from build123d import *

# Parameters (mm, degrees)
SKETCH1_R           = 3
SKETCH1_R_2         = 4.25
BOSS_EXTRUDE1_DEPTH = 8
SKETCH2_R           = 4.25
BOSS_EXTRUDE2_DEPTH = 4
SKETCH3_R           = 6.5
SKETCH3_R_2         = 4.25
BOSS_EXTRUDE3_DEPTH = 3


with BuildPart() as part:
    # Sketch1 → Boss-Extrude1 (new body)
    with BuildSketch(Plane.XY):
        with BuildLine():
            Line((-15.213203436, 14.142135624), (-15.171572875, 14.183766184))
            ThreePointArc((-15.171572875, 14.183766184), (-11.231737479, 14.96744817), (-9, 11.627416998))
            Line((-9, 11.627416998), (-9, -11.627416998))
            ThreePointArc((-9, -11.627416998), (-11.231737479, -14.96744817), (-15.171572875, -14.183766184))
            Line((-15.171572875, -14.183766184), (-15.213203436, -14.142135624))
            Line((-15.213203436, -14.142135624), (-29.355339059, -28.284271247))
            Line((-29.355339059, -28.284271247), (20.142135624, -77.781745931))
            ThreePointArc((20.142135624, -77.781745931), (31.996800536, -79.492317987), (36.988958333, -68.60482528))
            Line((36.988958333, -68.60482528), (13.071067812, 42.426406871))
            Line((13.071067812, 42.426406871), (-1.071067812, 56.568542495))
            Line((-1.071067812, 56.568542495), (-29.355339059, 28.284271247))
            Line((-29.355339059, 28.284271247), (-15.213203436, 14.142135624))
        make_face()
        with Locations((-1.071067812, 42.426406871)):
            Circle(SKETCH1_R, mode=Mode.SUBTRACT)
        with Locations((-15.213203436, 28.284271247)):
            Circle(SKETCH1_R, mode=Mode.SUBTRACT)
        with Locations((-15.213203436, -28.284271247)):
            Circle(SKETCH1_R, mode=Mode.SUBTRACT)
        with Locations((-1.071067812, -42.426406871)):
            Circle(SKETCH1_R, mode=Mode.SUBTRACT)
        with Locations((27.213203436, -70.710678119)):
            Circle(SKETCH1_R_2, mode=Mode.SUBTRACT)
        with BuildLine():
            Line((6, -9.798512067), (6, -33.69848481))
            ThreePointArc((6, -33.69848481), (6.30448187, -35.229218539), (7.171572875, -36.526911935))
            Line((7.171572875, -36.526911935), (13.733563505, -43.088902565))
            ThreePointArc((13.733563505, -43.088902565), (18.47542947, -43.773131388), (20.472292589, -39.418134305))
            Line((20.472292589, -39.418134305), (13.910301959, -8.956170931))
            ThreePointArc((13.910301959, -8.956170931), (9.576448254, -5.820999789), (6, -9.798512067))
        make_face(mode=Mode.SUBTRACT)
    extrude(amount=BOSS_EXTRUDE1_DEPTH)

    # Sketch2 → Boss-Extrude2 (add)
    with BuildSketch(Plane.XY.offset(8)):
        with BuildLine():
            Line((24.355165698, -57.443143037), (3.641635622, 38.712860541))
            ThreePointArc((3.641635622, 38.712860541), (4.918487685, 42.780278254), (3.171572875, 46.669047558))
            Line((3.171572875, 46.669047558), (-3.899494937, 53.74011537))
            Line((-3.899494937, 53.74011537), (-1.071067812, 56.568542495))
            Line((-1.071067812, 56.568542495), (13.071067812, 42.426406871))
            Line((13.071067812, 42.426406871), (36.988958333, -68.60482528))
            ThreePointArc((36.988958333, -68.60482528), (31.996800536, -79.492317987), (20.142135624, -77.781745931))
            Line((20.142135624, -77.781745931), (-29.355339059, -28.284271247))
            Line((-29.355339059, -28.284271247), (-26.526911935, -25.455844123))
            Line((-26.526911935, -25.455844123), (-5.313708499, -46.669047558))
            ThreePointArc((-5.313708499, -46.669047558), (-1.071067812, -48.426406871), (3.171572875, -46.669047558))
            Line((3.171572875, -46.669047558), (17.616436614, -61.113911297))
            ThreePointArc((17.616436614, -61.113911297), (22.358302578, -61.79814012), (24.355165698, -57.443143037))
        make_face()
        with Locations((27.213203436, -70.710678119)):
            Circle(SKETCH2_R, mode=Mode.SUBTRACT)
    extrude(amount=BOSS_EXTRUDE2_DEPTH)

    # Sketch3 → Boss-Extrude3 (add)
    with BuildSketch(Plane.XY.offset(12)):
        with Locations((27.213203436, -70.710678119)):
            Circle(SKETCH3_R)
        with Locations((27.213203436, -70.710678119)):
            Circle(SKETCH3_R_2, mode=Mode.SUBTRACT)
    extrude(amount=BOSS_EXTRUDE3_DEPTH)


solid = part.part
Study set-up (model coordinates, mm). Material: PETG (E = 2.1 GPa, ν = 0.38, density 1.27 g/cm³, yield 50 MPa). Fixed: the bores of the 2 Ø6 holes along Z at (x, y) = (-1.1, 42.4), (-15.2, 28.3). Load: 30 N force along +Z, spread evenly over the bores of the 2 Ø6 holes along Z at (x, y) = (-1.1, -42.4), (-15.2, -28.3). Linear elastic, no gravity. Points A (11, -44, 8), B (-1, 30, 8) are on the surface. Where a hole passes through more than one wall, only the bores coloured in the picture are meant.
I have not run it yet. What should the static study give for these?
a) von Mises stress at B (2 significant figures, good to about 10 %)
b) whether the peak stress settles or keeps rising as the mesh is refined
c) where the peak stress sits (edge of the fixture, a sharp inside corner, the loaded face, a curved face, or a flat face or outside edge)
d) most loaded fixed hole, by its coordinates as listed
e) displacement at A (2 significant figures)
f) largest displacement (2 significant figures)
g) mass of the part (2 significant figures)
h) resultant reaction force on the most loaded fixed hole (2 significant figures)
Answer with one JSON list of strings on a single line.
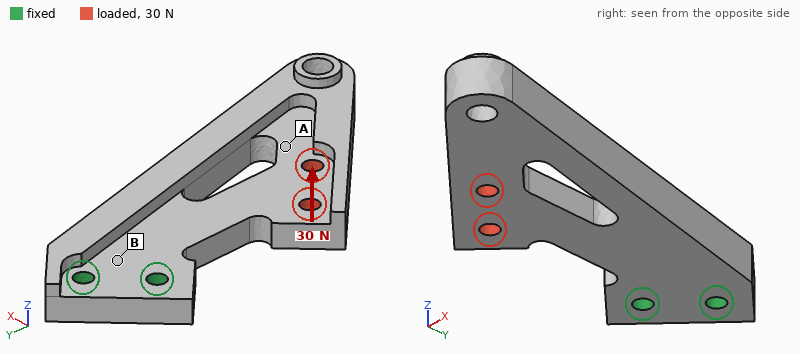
["2.2 MPa", "keeps rising", "edge of the fixture", "(-15.2, 28.3)", "0.90 mm", "1.4 mm", "52 g", "67 N"]
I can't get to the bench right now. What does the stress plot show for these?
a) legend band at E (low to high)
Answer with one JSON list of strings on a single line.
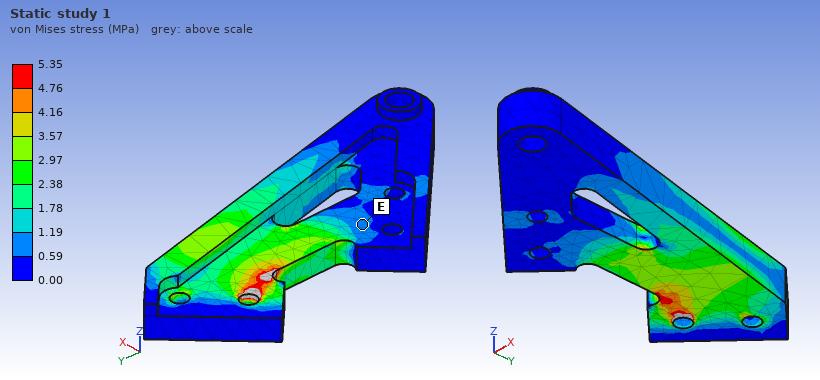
["0.59 to 1.19 MPa"]
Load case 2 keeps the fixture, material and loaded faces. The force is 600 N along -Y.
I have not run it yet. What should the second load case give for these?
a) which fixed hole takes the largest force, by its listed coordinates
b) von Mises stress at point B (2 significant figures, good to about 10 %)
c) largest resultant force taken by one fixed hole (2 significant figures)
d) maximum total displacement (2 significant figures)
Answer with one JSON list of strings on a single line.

["(-15.2, 28.3)", "3.6 MPa", "330 N", "0.94 mm"]
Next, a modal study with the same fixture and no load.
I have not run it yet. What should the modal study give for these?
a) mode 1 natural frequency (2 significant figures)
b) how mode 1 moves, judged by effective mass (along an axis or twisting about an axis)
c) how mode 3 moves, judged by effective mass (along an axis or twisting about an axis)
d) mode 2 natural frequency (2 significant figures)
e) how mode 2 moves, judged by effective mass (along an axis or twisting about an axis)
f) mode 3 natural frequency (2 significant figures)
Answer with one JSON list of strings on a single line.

["140 Hz", "along Z", "twisting about Y", "380 Hz", "along X", "480 Hz"]
